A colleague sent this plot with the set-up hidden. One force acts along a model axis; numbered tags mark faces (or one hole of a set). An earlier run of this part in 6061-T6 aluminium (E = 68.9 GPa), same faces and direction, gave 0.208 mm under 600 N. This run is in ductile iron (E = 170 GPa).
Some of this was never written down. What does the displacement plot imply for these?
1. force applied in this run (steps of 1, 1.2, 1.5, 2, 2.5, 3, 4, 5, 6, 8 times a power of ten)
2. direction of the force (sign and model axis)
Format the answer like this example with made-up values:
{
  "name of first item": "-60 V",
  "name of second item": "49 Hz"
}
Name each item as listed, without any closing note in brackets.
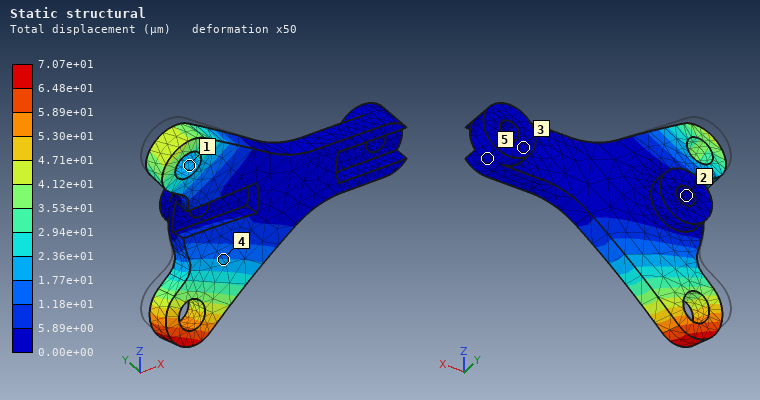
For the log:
{
  "force applied in this run": "500 N",
  "direction of the force": "-Y"
}
